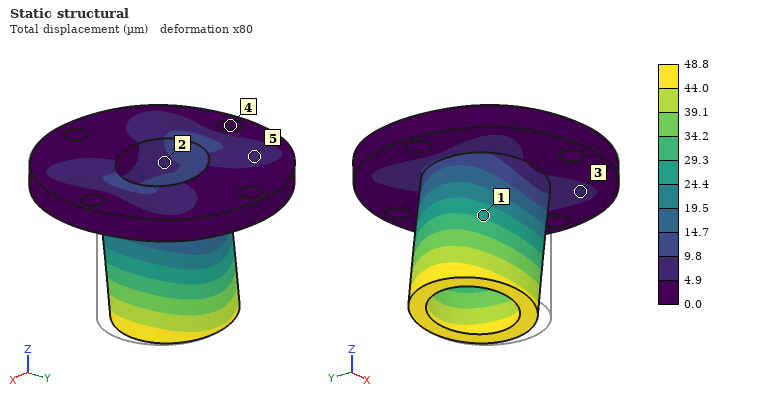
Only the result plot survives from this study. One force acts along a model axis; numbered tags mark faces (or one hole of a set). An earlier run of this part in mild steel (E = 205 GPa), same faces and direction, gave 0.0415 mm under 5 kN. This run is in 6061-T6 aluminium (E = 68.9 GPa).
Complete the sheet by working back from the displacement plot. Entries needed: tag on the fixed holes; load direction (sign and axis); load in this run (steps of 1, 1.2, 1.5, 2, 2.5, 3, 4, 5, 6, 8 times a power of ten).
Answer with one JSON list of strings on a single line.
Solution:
["4", "-X", "2 kN"]
